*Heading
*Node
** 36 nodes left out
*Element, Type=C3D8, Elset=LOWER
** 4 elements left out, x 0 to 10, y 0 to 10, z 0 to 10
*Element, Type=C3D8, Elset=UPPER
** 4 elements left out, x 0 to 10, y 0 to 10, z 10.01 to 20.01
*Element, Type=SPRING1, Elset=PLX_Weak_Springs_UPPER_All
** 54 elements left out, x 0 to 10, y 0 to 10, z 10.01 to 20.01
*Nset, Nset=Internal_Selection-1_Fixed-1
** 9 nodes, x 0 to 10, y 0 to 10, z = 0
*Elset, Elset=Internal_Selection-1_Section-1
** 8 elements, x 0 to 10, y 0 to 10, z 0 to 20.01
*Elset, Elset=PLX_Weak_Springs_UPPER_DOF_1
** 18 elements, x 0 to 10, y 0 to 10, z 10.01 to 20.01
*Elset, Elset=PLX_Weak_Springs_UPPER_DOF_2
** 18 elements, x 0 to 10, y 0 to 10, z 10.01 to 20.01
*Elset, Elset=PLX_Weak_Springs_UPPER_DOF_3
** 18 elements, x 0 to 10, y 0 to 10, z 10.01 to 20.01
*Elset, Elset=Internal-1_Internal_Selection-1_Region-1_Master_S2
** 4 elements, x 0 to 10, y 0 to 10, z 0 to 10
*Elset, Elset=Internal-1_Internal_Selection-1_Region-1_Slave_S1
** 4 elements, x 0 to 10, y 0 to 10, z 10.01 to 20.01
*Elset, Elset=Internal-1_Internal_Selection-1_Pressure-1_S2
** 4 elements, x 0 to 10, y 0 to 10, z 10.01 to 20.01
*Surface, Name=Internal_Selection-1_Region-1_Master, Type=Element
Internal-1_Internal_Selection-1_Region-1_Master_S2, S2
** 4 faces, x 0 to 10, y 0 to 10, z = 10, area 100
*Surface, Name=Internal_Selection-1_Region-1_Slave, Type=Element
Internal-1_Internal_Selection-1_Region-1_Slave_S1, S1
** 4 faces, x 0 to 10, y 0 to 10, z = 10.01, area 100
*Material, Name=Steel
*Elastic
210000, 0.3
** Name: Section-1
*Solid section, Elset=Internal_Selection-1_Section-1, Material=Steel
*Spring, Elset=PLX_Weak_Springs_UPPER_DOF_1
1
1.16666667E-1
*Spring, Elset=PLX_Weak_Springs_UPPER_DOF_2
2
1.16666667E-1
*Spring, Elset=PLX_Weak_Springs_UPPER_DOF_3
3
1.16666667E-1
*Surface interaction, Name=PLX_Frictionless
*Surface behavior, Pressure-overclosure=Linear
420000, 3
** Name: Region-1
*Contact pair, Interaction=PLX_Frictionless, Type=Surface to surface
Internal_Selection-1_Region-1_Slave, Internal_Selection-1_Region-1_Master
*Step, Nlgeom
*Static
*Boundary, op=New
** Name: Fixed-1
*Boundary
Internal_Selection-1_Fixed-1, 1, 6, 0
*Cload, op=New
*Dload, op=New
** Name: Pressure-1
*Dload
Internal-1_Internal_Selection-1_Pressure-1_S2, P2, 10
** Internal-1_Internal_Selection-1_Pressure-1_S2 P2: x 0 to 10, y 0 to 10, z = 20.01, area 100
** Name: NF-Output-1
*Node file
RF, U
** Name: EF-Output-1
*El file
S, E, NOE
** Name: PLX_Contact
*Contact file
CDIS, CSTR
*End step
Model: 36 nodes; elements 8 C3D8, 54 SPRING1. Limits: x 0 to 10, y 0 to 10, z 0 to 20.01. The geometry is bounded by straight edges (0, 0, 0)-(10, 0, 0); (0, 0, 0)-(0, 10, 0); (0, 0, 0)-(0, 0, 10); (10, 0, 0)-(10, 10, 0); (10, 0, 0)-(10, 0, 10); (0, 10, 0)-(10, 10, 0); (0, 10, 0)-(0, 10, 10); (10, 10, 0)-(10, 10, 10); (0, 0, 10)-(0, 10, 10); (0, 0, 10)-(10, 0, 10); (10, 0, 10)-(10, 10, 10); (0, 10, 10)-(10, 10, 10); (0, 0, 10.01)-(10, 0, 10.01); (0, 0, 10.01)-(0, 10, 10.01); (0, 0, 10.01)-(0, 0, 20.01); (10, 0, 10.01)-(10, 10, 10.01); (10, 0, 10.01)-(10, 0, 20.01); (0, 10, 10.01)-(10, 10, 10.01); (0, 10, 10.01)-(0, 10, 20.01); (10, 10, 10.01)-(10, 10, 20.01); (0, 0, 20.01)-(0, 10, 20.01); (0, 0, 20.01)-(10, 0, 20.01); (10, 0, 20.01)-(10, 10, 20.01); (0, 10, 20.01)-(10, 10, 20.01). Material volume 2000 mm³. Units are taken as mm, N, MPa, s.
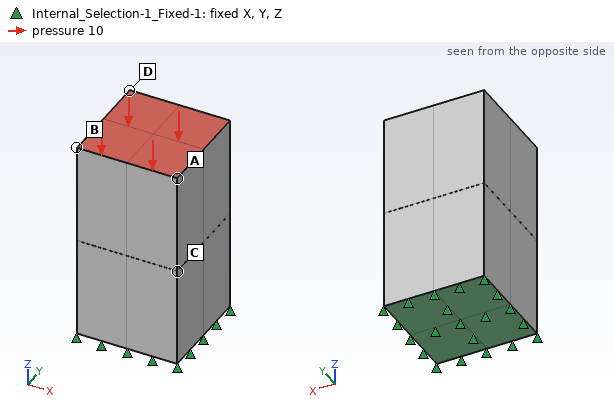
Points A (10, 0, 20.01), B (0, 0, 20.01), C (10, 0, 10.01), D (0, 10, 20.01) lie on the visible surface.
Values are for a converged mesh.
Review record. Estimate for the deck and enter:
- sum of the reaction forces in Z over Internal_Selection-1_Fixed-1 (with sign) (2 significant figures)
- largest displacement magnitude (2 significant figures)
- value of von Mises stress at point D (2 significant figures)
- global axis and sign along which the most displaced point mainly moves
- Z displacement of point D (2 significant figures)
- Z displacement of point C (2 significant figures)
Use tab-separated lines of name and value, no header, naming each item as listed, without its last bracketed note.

sum of the reaction forces in Z over Internal_Selection-1_Fixed-1 (with sign)	1000 N
largest displacement magnitude	0.011 mm
value of von Mises stress at point D	10 MPa
global axis and sign along which the most displaced point mainly moves	-Z
Z displacement of point D	-0.011 mm
Z displacement of point C	-0.010 mm
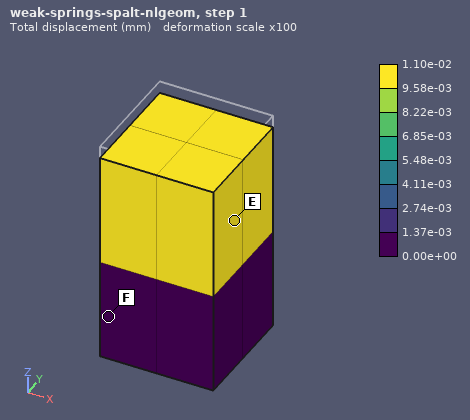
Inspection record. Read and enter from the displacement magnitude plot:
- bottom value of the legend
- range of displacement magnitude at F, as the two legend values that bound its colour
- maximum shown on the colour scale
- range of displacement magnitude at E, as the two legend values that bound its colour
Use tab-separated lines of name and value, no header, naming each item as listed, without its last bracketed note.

bottom value of the legend	0.00e+00 mm
range of displacement magnitude at F, as the two legend values that bound its colour	0.00e+00 to 1.37e-03 mm
maximum shown on the colour scale	1.10e-02 mm
range of displacement magnitude at E, as the two legend values that bound its colour	9.58e-03 to 1.10e-02 mm
